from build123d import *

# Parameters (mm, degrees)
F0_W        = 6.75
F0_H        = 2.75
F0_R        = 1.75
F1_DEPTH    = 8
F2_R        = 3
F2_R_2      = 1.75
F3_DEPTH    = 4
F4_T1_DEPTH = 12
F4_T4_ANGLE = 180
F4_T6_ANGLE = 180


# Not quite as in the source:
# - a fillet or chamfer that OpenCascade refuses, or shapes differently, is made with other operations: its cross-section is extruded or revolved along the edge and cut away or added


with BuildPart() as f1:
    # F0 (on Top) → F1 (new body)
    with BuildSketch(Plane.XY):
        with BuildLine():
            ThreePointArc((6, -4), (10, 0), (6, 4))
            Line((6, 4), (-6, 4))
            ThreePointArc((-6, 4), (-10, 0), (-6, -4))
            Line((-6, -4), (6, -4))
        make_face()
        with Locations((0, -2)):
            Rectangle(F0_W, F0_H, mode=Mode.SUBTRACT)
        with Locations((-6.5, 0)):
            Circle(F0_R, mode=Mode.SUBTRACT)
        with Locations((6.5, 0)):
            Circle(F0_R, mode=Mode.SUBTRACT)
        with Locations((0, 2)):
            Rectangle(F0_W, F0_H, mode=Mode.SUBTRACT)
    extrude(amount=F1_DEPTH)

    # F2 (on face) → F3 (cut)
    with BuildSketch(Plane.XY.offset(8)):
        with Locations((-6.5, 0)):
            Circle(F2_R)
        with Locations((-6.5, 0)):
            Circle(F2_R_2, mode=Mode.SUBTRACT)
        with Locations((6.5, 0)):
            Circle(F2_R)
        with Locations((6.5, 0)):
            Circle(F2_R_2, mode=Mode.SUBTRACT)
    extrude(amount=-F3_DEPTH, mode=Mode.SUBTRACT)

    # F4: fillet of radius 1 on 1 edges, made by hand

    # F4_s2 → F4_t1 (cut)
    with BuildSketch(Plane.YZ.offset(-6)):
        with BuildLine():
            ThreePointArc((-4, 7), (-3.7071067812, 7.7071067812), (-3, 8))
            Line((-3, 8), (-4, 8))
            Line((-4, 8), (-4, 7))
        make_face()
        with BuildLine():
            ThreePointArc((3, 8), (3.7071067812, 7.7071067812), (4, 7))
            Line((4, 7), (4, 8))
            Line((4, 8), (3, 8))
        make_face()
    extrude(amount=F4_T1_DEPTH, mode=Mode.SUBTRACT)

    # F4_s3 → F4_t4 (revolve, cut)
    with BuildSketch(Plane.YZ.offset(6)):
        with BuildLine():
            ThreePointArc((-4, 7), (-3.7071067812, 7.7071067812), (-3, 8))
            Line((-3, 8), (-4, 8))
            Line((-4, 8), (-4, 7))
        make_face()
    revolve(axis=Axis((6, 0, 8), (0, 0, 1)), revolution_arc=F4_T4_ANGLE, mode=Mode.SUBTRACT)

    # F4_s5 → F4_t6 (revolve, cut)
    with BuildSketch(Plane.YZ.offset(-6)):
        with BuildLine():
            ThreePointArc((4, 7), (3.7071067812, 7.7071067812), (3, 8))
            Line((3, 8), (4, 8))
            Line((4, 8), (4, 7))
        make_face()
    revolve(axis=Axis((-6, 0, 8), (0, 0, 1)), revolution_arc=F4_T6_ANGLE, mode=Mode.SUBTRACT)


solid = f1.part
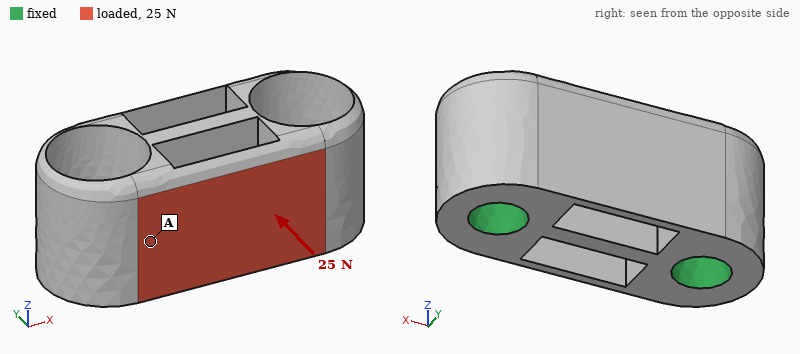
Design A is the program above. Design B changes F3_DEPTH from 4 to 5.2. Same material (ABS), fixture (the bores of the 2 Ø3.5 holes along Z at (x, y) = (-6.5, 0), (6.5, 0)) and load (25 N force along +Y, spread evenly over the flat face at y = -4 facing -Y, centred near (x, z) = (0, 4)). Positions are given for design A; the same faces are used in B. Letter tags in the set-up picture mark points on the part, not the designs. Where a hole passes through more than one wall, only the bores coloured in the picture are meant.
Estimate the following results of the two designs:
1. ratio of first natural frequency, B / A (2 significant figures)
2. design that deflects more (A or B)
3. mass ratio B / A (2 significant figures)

0.82
B
0.92
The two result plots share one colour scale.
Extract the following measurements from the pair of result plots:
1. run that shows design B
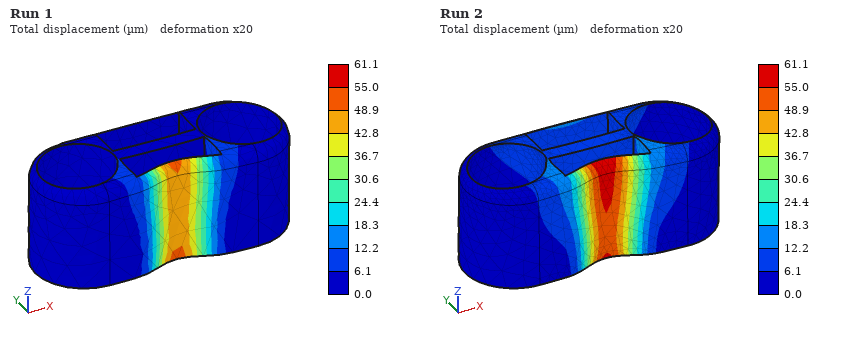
Run 2
